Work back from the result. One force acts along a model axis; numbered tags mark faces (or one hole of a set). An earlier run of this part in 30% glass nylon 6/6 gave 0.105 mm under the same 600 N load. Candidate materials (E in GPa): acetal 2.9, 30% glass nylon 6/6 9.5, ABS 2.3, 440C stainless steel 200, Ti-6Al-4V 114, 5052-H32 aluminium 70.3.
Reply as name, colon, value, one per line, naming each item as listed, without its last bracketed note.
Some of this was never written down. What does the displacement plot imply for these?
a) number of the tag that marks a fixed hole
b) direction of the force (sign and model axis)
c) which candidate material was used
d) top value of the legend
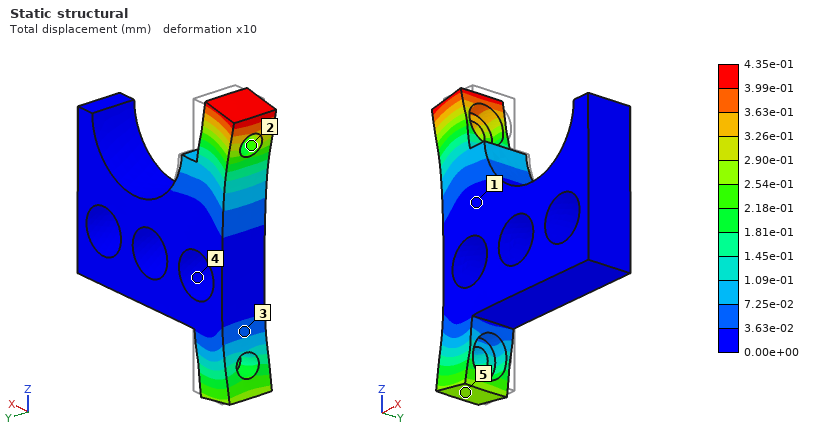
number of the tag that marks a fixed hole: 4
direction of the force: -X
which candidate material was used: ABS
top value of the legend: 4.35e-01 mm
